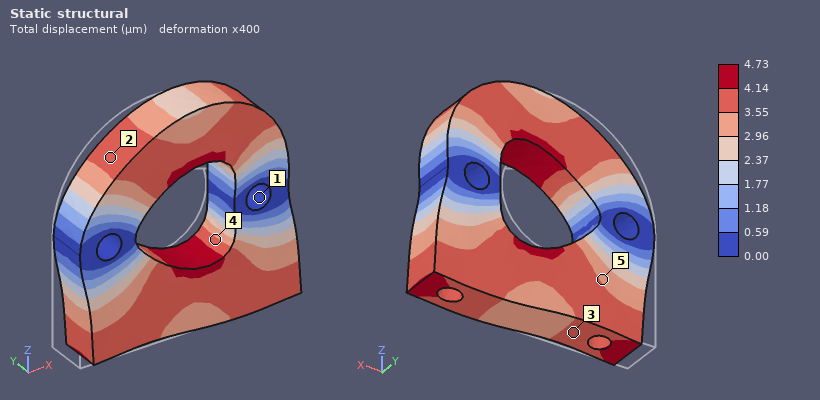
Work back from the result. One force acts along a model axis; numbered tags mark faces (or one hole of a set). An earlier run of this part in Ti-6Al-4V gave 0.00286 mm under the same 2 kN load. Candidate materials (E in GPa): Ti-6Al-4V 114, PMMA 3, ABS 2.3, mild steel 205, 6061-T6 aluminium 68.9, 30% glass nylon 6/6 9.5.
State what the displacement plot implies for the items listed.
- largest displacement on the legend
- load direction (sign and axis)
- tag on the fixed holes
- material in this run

4.73 µm
+X
1
6061-T6 aluminium
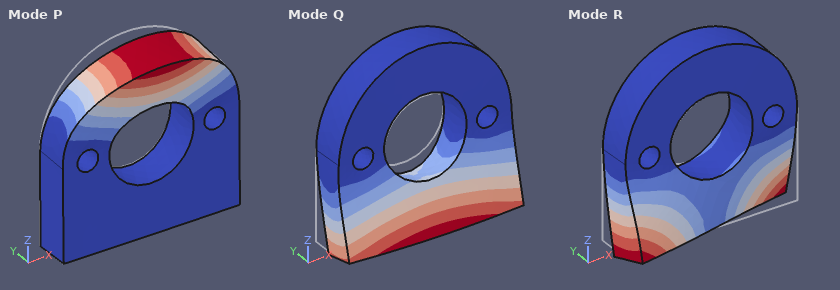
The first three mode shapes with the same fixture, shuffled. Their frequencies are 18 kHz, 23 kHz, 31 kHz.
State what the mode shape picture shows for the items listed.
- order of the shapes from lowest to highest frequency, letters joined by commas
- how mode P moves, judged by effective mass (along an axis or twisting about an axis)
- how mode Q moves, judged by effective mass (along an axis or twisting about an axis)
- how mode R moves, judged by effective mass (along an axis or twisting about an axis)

Q, P, R
along Y
along Y
twisting about Z
